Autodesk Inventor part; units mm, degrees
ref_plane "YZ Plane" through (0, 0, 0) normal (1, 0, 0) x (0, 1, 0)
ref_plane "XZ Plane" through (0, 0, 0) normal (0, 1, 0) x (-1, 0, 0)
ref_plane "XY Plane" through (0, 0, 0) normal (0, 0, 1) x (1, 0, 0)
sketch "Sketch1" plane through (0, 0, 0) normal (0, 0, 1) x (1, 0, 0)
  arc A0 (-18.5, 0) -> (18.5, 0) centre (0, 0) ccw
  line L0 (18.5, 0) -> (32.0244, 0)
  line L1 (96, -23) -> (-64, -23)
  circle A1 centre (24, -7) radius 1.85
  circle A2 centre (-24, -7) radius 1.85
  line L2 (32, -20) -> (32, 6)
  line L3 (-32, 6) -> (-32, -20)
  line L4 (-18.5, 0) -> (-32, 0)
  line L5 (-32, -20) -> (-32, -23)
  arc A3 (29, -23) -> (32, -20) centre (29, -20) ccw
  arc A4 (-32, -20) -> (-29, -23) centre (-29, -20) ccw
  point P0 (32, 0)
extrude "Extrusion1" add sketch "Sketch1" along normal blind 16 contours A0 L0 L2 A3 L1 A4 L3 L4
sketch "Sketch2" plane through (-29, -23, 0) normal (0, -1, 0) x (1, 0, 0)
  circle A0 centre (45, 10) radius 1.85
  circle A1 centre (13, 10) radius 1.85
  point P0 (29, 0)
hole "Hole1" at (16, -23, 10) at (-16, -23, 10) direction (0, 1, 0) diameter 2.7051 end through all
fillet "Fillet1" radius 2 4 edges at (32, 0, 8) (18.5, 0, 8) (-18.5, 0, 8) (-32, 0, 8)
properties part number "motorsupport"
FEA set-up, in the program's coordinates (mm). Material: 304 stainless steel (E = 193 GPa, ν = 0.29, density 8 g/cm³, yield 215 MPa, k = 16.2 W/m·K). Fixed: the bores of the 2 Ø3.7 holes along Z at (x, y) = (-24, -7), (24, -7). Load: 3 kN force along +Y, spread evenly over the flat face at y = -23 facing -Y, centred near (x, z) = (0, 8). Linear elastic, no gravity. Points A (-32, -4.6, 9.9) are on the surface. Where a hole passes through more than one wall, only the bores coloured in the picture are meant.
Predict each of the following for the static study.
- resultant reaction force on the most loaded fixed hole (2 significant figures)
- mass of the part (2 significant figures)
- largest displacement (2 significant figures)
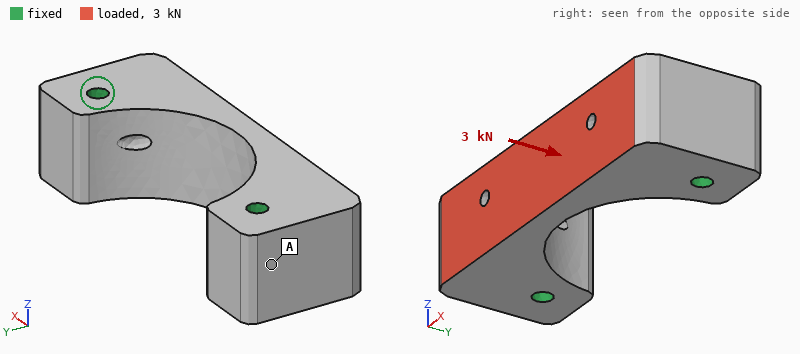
1.7 kN
110 g
3.5 µm
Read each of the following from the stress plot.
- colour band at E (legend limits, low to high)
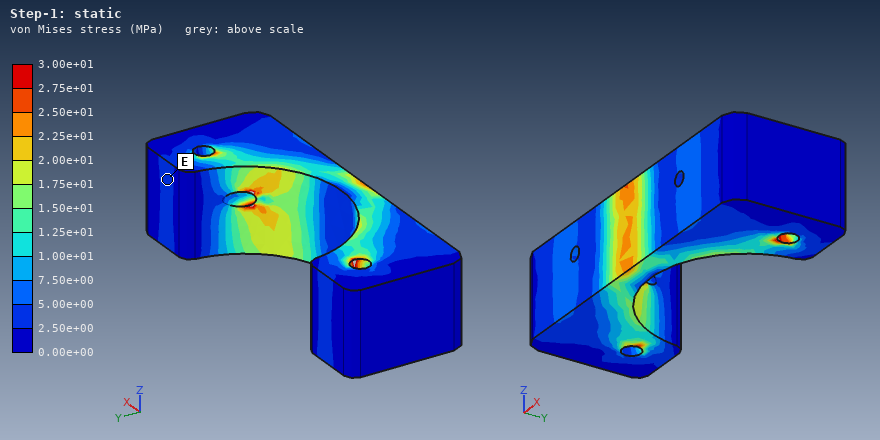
2.50e+00 to 5.00e+00 MPa
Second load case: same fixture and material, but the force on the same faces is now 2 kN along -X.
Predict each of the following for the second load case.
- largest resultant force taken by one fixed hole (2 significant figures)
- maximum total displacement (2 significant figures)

1.1 kN
3.0 µm
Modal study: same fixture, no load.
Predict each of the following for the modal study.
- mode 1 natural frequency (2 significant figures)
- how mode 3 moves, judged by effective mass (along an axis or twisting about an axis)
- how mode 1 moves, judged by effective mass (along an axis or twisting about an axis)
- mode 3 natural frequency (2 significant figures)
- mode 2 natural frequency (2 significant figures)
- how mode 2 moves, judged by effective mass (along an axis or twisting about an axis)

17 kHz
along Y
along X
25 kHz
18 kHz
along Z
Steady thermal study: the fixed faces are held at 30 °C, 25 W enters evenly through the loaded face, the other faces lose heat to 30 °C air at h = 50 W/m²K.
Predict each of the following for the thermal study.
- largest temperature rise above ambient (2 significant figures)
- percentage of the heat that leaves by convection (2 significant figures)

66 K
18 %
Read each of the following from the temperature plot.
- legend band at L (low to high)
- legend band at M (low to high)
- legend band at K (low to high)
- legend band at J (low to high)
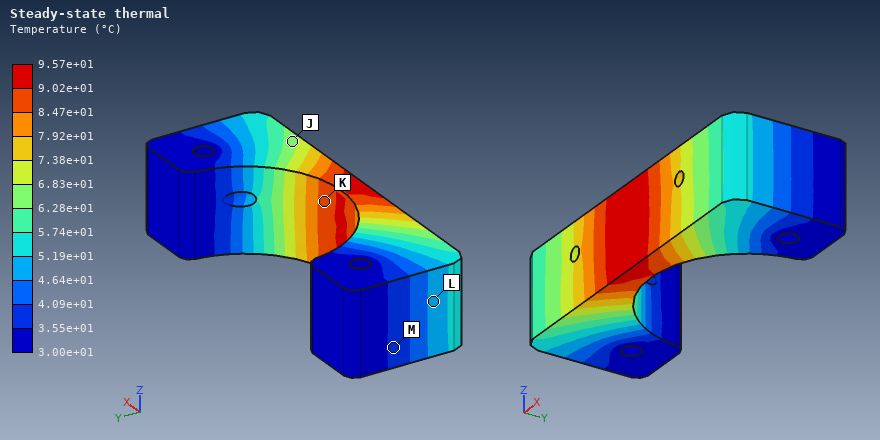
4.64e+01 to 5.19e+01 °C
3.55e+01 to 4.09e+01 °C
8.47e+01 to 9.02e+01 °C
6.28e+01 to 6.83e+01 °C
